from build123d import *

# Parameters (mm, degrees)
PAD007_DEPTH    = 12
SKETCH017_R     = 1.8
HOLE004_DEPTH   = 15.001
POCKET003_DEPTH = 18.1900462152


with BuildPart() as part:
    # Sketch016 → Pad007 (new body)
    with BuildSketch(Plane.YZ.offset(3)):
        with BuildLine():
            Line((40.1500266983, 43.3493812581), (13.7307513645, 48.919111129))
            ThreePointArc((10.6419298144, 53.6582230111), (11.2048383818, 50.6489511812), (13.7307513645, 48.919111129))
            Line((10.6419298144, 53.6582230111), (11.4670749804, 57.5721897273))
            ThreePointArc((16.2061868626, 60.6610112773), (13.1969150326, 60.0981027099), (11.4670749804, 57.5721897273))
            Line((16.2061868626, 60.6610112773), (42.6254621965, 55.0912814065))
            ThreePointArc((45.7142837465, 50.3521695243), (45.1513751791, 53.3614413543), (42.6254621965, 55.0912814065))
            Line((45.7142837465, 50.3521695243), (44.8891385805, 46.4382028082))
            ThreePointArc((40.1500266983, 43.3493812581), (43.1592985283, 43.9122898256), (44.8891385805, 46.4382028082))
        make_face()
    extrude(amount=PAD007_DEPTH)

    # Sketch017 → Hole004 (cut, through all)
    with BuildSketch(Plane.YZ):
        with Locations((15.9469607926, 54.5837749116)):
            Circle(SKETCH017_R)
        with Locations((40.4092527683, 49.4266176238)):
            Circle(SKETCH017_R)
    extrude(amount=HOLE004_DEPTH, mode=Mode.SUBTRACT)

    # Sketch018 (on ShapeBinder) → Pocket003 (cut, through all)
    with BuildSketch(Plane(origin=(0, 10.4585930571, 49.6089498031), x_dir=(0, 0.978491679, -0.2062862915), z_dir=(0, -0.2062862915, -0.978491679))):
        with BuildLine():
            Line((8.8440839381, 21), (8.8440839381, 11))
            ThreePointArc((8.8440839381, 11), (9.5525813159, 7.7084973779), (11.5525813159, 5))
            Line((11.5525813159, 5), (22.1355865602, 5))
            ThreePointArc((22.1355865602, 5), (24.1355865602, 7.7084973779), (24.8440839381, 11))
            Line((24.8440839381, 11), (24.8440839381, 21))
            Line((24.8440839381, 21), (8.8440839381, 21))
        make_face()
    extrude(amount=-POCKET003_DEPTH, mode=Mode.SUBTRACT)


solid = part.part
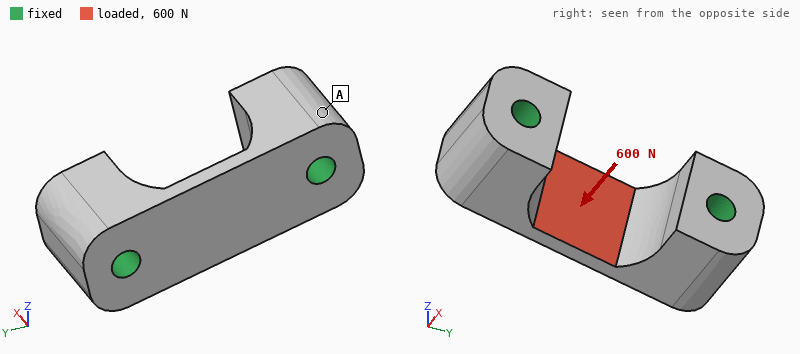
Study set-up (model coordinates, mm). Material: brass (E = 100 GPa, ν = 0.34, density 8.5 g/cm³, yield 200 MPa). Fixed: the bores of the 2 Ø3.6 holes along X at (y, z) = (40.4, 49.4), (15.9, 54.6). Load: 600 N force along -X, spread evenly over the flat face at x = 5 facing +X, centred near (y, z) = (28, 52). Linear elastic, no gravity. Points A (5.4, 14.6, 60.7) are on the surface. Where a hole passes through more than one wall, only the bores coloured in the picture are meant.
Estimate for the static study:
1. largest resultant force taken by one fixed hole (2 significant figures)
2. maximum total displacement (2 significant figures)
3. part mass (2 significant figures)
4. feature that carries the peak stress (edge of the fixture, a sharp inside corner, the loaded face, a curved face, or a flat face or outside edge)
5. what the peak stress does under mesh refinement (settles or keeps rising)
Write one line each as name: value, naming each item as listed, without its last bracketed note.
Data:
largest resultant force taken by one fixed hole: 350 N
maximum total displacement: 8.9 µm
part mass: 24 g
feature that carries the peak stress: a sharp inside corner
what the peak stress does under mesh refinement: keeps rising
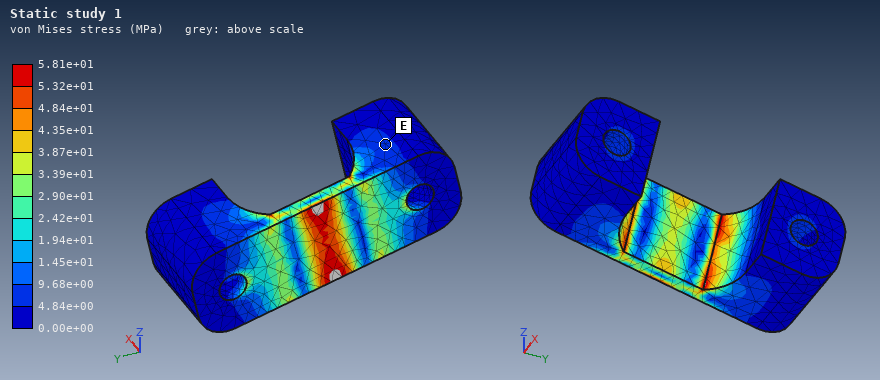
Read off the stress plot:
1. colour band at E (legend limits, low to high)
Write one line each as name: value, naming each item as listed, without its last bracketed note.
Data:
colour band at E: 4.84e+00 to 9.68e+00 MPa
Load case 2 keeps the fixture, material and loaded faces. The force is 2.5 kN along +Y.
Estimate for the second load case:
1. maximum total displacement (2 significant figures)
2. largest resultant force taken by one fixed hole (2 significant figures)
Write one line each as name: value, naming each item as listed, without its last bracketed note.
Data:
maximum total displacement: 7.8 µm
largest resultant force taken by one fixed hole: 1.3 kN
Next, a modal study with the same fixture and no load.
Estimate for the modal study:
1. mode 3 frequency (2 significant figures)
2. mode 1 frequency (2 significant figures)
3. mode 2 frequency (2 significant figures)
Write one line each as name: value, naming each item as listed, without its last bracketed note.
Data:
mode 3 frequency: 40 kHz
mode 1 frequency: 32 kHz
mode 2 frequency: 36 kHz
